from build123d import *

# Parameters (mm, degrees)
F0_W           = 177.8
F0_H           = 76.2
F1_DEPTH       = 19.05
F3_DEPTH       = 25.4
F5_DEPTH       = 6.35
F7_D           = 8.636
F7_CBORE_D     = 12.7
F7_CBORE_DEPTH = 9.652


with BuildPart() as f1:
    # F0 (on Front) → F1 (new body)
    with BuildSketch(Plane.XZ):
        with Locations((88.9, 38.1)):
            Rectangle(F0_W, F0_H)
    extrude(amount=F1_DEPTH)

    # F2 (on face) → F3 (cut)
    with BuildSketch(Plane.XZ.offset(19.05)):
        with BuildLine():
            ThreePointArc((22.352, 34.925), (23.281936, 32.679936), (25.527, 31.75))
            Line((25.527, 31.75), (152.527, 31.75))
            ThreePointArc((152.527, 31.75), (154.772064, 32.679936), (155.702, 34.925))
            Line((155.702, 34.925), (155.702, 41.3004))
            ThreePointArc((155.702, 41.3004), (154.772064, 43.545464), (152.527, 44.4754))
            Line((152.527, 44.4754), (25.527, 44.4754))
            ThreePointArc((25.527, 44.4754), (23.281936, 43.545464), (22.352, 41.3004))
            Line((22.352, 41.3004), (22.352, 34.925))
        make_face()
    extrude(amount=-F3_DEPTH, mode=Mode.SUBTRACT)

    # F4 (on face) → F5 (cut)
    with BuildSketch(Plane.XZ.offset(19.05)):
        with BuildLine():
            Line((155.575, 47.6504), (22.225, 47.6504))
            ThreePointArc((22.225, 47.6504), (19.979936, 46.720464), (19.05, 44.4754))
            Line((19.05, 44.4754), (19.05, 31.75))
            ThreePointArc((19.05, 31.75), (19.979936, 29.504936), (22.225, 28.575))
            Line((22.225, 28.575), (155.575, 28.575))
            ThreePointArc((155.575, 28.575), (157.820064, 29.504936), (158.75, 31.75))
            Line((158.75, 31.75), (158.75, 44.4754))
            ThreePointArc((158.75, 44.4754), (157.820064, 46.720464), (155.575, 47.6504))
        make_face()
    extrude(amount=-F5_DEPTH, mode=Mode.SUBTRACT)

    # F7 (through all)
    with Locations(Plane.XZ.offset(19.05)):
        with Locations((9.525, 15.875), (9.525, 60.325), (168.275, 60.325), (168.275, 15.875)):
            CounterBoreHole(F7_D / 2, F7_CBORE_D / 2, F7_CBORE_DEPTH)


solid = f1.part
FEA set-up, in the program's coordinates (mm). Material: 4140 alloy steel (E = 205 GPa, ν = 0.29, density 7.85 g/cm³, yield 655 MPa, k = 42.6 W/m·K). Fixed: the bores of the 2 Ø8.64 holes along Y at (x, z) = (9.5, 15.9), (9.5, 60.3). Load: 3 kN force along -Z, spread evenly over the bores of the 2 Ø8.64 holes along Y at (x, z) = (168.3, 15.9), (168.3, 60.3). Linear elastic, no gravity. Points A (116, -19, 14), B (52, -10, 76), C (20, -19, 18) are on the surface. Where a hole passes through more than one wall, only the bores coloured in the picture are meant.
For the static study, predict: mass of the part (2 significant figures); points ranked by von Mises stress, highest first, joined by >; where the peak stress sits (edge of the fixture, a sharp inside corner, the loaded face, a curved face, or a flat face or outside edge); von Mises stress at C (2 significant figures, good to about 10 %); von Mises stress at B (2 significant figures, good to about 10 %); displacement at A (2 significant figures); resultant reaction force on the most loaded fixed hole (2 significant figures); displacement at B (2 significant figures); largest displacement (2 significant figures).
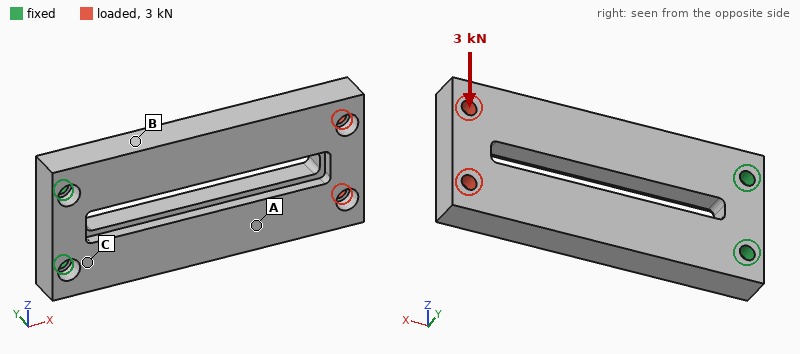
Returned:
1.7 kg
B > C > A
edge of the fixture
24 MPa
32 MPa
0.067 mm
8.9 kN
0.024 mm
0.11 mm
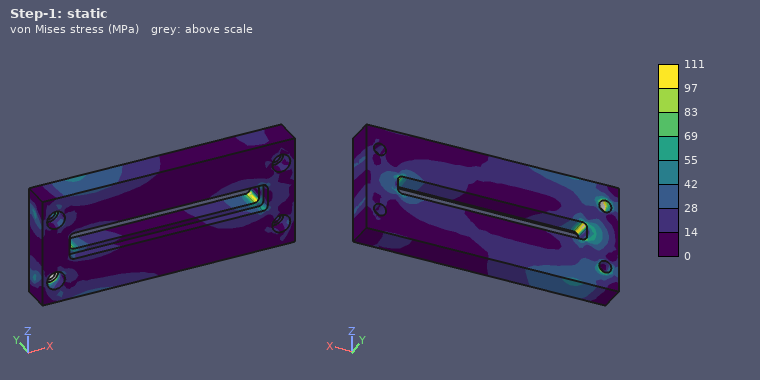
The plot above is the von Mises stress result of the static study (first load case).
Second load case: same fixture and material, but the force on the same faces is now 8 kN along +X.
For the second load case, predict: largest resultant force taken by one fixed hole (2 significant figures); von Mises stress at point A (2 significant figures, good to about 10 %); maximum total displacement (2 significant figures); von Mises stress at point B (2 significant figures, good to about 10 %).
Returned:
4.0 kN
3.5 MPa
69 µm
6.2 MPa
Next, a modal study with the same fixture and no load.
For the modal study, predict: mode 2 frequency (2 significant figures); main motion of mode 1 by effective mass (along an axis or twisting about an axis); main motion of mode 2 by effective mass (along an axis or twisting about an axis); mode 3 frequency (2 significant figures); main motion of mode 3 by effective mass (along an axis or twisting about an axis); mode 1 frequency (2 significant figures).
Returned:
1100 Hz
along Y
along Z
1700 Hz
twisting about X
430 Hz
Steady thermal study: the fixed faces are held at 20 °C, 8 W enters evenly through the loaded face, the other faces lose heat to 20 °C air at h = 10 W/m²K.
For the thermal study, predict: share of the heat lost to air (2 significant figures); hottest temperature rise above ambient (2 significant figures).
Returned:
43 %
20 K
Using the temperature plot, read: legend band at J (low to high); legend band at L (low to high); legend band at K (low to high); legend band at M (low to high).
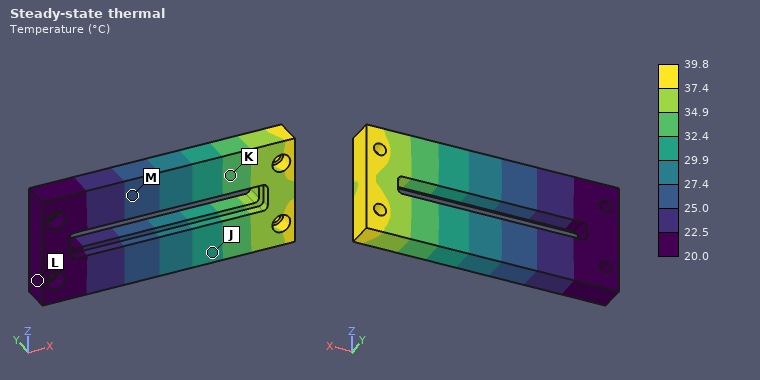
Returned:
29.9 to 32.4 °C
20.0 to 22.5 °C
32.4 to 34.9 °C
25.0 to 27.4 °C
